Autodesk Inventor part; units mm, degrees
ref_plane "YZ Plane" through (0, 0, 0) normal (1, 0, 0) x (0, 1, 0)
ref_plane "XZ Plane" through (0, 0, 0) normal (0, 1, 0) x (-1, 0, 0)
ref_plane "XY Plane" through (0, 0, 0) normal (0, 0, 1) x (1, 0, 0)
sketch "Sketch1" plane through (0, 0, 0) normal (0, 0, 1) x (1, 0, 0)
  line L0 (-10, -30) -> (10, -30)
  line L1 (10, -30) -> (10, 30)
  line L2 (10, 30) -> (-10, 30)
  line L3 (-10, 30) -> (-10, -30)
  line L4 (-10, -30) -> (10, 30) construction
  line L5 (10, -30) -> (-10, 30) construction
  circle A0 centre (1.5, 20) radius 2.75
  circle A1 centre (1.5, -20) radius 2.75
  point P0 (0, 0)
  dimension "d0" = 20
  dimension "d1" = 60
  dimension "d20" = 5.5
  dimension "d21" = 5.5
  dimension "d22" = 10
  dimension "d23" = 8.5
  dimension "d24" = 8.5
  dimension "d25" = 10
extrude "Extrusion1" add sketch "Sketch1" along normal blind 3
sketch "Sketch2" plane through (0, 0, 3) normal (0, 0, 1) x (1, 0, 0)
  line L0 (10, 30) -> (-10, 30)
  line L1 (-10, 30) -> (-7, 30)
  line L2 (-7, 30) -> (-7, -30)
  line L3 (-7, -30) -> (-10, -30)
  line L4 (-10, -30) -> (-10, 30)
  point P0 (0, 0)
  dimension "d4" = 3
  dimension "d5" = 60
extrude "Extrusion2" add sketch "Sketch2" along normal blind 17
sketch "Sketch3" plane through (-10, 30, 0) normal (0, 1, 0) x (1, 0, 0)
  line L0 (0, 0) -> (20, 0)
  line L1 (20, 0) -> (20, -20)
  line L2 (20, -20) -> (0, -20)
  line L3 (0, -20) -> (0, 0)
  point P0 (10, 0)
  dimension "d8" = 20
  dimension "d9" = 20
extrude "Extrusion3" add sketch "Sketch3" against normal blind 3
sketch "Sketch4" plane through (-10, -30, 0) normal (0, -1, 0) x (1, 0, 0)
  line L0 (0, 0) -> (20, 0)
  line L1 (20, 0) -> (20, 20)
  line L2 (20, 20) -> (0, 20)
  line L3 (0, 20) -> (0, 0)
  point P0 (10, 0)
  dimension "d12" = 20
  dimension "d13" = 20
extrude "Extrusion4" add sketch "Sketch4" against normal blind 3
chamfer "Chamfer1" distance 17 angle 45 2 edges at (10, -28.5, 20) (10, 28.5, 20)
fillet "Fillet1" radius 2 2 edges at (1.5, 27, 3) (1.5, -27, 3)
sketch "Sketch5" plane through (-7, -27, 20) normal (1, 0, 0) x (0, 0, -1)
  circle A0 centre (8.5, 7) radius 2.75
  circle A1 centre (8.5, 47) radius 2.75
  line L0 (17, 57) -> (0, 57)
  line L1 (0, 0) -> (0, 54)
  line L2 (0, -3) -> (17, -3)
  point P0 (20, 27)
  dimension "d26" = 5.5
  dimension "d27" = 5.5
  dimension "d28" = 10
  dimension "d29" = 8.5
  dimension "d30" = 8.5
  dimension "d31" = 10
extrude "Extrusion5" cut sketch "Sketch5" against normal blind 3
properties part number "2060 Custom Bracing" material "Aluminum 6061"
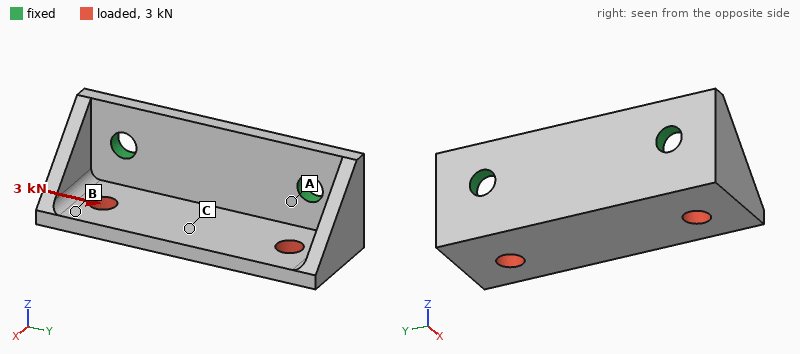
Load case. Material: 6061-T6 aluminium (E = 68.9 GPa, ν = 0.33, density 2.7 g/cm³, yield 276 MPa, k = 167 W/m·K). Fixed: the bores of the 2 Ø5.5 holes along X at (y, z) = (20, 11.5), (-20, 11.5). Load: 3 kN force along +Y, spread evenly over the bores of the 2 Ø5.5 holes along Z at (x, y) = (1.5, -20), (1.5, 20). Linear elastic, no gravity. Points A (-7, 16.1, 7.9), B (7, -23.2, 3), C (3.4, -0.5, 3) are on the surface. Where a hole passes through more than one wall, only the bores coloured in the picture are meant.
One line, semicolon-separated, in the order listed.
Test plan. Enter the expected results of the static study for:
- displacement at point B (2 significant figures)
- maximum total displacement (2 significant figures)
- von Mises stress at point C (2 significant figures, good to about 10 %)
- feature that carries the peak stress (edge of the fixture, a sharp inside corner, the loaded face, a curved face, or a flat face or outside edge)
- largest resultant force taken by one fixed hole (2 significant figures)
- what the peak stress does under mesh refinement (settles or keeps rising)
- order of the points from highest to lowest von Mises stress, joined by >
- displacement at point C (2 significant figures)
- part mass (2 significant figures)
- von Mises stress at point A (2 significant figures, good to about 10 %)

74 µm; 95 µm; 39 MPa; edge of the fixture; 1.8 kN; keeps rising; A > C > B; 36 µm; 20 g; 79 MPa
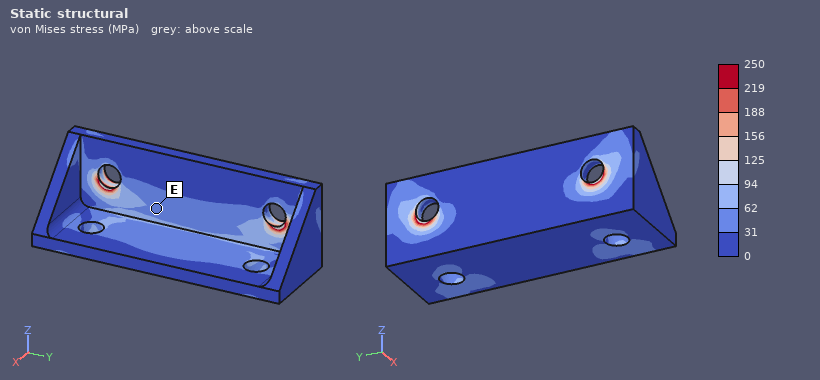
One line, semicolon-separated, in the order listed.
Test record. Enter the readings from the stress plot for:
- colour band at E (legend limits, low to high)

31 to 62 MPa
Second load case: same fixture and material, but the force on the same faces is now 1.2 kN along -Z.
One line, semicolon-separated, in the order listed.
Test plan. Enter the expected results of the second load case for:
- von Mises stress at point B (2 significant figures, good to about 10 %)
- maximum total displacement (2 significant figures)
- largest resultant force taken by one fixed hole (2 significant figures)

22 MPa; 0.15 mm; 610 N
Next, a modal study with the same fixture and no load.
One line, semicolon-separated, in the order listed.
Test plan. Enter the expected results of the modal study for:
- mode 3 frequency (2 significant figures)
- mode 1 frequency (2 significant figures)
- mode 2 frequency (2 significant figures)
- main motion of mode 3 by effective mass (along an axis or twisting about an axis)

10 kHz; 5200 Hz; 7200 Hz; along X
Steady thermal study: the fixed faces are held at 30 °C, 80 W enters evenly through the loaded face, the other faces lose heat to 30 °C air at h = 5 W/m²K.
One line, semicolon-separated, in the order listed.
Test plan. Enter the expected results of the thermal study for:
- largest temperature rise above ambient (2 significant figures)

61 K
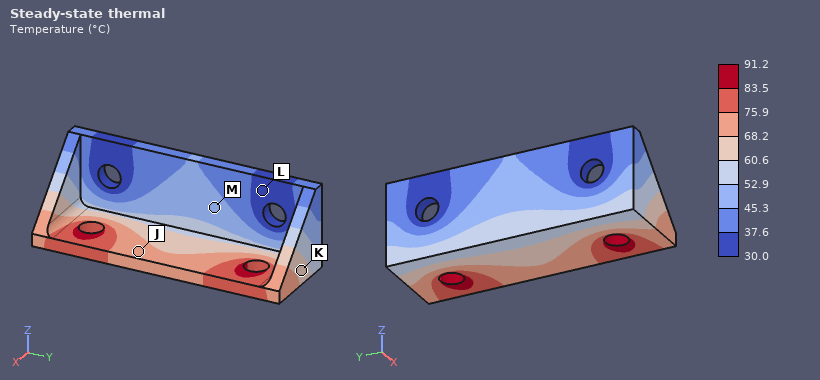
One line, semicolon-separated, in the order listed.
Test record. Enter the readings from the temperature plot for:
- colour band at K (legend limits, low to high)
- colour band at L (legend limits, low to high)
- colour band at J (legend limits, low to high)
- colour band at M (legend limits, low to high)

60.6 to 68.2 °C; 30.0 to 37.6 °C; 68.2 to 75.9 °C; 45.3 to 52.9 °C
